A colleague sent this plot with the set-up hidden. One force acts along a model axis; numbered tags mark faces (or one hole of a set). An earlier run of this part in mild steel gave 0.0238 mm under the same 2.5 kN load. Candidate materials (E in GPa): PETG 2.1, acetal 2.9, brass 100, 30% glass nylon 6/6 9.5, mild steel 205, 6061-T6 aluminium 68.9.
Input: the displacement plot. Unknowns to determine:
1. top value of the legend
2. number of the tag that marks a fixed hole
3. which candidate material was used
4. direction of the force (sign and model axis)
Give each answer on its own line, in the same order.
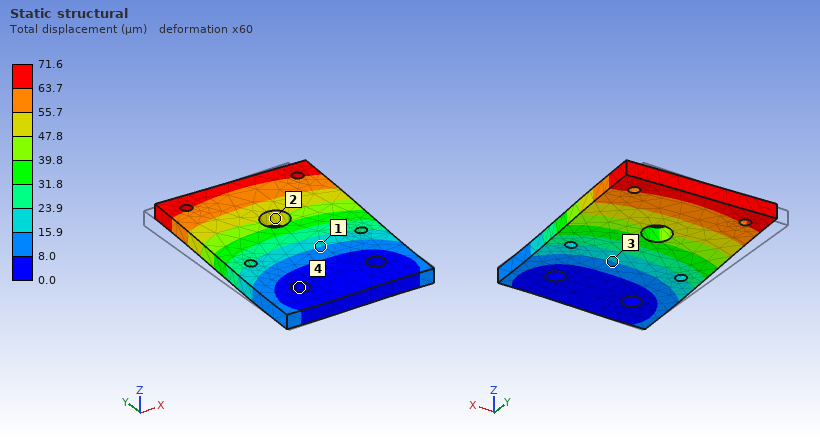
71.6 µm
4
6061-T6 aluminium
+X
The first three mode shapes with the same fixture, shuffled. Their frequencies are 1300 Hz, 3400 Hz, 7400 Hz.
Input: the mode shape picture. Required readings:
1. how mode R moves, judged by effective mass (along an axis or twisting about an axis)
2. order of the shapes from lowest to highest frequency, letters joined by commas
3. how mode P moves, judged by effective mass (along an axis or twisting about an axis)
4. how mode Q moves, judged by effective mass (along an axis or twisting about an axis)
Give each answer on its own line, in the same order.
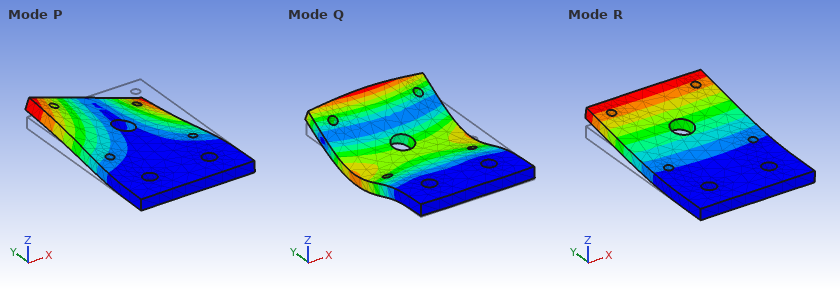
along Z
R, P, Q
twisting about Y
along Z
